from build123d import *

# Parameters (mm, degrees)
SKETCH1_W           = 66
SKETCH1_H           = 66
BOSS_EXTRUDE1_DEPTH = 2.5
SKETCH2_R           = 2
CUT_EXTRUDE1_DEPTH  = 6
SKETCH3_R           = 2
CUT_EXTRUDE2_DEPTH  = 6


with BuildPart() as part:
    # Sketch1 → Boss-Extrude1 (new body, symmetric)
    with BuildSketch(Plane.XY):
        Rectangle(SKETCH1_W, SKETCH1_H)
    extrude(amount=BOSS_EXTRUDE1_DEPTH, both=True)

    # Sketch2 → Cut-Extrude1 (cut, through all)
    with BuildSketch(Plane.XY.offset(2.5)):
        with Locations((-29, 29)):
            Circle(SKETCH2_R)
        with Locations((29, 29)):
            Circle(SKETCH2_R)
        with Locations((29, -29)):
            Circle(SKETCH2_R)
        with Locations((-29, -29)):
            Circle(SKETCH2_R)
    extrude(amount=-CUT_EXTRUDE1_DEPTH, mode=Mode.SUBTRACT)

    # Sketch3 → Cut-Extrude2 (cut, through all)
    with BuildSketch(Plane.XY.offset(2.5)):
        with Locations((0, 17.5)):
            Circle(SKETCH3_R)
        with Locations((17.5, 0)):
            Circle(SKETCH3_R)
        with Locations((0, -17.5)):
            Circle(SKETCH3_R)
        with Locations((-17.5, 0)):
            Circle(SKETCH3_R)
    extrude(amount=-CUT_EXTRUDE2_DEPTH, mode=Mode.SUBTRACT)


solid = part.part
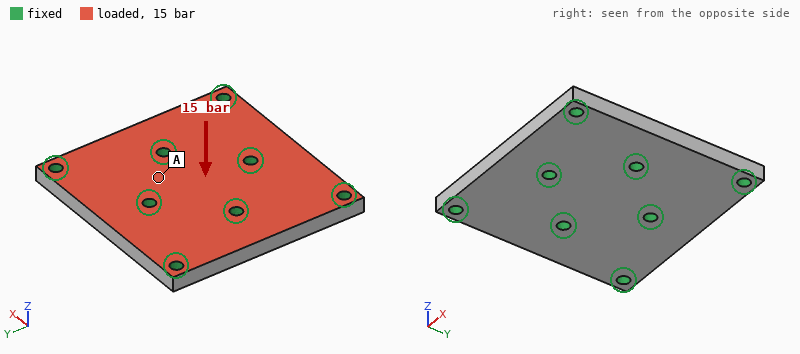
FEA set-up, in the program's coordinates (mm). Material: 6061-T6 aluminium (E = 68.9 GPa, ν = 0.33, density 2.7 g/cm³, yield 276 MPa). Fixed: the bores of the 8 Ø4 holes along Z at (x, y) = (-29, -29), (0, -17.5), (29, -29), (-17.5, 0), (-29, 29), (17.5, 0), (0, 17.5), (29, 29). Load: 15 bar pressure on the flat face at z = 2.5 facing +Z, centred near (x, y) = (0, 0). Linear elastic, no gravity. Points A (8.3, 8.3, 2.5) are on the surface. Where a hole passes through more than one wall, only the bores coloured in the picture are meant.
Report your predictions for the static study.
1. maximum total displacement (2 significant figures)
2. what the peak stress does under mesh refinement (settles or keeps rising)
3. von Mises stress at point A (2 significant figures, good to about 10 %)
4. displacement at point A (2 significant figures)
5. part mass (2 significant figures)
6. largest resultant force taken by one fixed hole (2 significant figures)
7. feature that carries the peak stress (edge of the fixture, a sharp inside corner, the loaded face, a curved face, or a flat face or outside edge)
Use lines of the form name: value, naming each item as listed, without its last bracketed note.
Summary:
maximum total displacement: 13 µm
what the peak stress does under mesh refinement: keeps rising
von Mises stress at point A: 10.0 MPa
displacement at point A: 3.1 µm
part mass: 57 g
largest resultant force taken by one fixed hole: 1.1 kN
feature that carries the peak stress: edge of the fixture
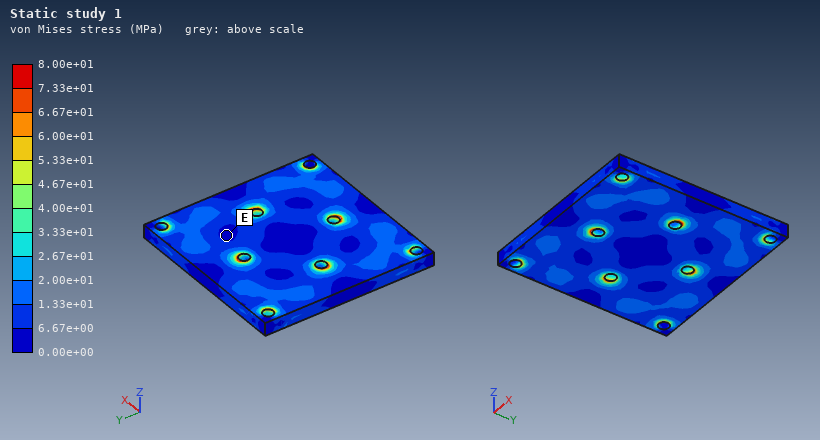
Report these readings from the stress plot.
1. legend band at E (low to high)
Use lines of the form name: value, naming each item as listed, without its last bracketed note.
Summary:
legend band at E: 0.00e+00 to 6.67e+00 MPa
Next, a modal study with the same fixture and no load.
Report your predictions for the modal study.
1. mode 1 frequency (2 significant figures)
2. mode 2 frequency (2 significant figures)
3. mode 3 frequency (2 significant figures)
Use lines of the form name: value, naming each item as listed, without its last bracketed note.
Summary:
mode 1 frequency: 17 kHz
mode 2 frequency: 18 kHz
mode 3 frequency: 18 kHz
